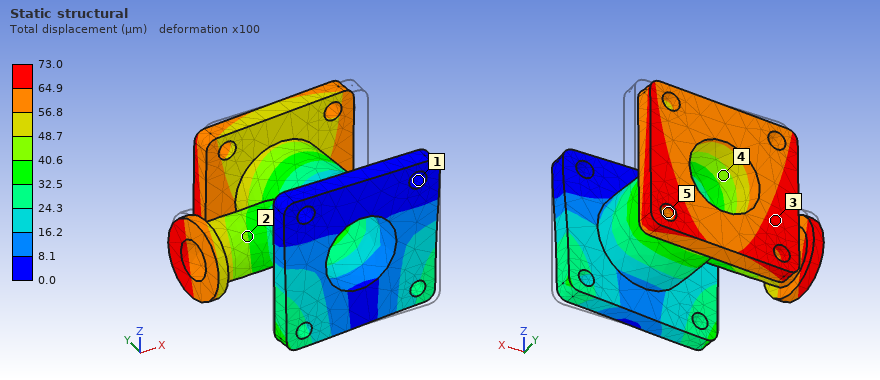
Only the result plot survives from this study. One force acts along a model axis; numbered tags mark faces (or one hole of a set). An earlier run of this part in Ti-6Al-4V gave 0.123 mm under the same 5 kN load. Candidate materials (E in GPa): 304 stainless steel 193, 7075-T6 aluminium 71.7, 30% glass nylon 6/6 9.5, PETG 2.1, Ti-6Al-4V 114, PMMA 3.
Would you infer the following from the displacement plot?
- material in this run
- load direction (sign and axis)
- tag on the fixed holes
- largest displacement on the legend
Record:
304 stainless steel
-X
1
73.0 µm
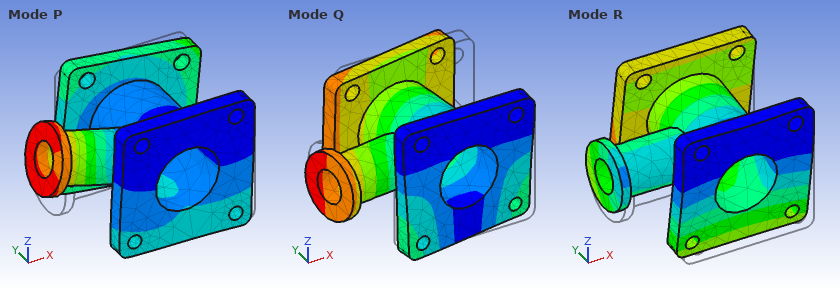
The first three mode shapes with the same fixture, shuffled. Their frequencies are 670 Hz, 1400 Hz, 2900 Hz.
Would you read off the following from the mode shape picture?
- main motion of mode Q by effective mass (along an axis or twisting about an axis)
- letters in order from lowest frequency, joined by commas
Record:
along X
R, Q, P
